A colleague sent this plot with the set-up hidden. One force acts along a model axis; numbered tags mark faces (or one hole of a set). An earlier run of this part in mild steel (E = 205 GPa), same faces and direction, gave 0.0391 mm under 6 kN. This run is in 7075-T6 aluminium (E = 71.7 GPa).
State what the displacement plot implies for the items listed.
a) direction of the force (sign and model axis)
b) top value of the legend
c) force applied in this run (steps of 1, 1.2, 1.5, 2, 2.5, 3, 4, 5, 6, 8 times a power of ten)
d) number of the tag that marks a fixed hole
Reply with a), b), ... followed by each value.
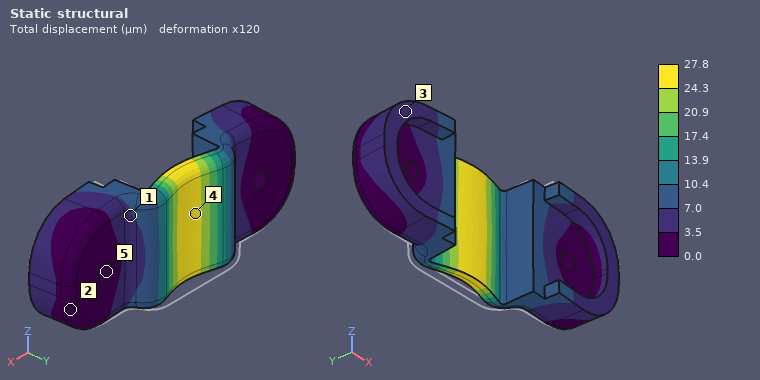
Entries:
a) -Y
b) 27.8 µm
c) 1.5 kN
d) 5
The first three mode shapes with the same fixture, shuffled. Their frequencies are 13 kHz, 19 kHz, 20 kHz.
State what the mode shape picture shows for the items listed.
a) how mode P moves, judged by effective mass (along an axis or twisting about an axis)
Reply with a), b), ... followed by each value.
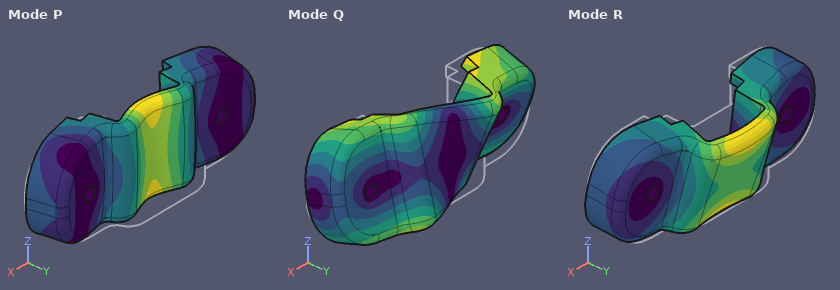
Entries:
a) along Y
